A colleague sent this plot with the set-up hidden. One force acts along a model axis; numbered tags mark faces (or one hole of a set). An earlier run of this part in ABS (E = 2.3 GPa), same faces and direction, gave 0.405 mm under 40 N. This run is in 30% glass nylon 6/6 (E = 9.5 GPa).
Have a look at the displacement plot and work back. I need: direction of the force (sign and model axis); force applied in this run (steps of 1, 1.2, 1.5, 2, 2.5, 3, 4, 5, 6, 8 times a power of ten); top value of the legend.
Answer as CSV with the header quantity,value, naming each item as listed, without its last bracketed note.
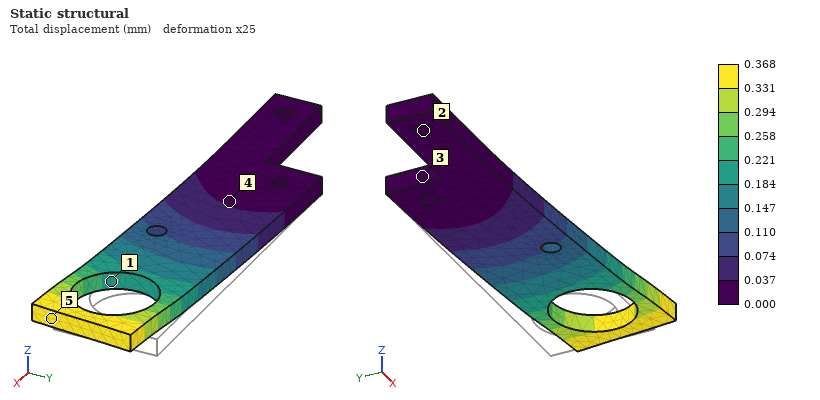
quantity,value
direction of the force,-Y
force applied in this run,150 N
top value of the legend,0.368 mm
